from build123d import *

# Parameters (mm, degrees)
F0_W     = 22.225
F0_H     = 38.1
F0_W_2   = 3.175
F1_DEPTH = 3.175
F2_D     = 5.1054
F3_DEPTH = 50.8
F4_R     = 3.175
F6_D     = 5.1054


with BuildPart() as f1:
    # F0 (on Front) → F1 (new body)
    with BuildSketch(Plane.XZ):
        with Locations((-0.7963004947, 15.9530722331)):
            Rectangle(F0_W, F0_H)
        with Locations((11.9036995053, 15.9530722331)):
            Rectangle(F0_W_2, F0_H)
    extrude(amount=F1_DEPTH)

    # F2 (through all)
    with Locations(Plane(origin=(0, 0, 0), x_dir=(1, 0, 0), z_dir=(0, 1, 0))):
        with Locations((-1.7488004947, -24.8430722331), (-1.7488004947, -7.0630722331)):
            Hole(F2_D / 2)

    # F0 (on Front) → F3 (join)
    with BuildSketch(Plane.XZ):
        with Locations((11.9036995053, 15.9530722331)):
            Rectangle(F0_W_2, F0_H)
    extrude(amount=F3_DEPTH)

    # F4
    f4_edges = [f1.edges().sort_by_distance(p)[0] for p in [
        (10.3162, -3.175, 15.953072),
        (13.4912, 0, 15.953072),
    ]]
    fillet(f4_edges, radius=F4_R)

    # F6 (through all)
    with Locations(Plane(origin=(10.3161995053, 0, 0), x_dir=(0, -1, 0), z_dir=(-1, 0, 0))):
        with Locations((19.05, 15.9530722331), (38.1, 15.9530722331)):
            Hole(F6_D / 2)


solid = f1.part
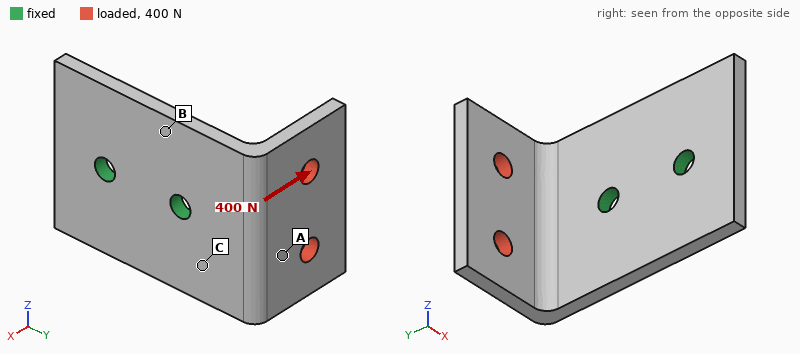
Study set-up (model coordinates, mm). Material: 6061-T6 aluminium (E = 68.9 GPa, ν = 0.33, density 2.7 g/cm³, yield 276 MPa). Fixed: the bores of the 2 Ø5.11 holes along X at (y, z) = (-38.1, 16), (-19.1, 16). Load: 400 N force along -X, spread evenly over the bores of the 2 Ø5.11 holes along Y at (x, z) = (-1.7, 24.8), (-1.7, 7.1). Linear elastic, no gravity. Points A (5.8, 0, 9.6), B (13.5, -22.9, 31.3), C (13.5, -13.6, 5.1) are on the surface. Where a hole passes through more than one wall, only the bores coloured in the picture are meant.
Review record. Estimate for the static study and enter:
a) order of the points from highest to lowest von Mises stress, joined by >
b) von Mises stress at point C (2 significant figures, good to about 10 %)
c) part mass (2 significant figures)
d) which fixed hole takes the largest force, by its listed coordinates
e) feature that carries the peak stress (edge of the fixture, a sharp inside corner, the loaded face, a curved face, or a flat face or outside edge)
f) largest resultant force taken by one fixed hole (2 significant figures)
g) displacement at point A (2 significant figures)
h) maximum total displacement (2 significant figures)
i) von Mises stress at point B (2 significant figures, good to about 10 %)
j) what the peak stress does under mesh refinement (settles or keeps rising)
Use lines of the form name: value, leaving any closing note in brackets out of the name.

order of the points from highest to lowest von Mises stress, joined by >: C > B > A
von Mises stress at point C: 55 MPa
part mass: 23 g
which fixed hole takes the largest force, by its listed coordinates: (-19.1, 16)
feature that carries the peak stress: edge of the fixture
largest resultant force taken by one fixed hole: 520 N
displacement at point A: 0.14 mm
maximum total displacement: 0.24 mm
von Mises stress at point B: 31 MPa
what the peak stress does under mesh refinement: keeps rising
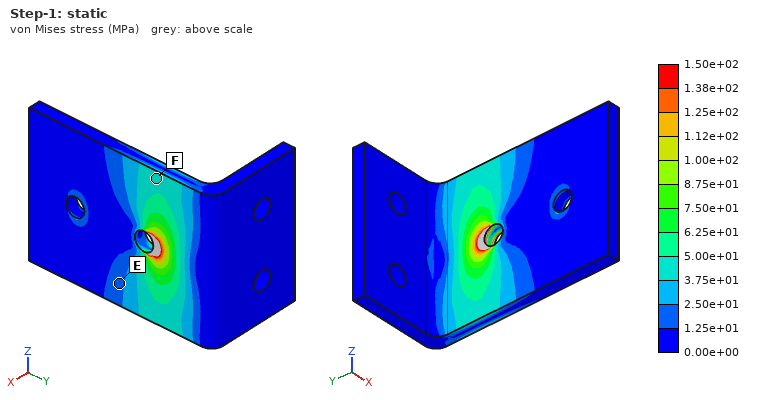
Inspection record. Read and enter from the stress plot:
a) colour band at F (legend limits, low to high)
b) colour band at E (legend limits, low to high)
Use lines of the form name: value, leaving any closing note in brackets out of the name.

colour band at F: 3.75e+01 to 5.00e+01 MPa
colour band at E: 1.25e+01 to 2.50e+01 MPa
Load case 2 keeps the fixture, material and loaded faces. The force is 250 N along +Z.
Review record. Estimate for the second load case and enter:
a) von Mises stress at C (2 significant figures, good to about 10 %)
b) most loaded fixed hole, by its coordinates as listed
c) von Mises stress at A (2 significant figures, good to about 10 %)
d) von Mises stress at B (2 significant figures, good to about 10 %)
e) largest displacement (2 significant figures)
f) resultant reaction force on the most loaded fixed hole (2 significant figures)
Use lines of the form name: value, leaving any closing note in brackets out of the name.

von Mises stress at C: 17 MPa
most loaded fixed hole, by its coordinates as listed: (-19.1, 16)
von Mises stress at A: 9.7 MPa
von Mises stress at B: 25 MPa
largest displacement: 0.14 mm
resultant reaction force on the most loaded fixed hole: 420 N
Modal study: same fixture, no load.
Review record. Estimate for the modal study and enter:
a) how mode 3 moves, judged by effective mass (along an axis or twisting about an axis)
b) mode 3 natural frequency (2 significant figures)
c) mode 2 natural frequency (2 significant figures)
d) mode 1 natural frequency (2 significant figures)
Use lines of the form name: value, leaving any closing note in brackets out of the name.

how mode 3 moves, judged by effective mass: along X
mode 3 natural frequency: 5900 Hz
mode 2 natural frequency: 2700 Hz
mode 1 natural frequency: 2100 Hz
